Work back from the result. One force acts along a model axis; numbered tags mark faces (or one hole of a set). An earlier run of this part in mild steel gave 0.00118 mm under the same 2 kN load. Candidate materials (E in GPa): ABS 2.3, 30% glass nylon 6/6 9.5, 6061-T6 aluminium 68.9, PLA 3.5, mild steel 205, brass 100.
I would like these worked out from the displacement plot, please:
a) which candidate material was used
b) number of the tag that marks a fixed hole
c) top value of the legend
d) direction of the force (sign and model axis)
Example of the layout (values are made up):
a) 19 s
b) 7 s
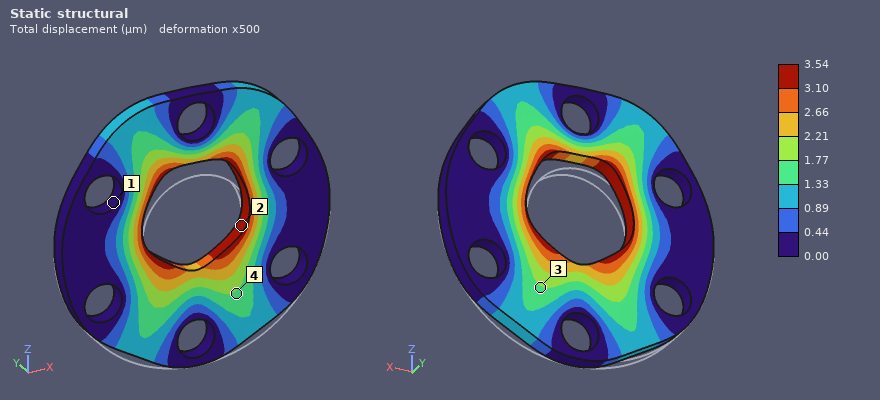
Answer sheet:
a) 6061-T6 aluminium
b) 1
c) 3.54 µm
d) +Z
